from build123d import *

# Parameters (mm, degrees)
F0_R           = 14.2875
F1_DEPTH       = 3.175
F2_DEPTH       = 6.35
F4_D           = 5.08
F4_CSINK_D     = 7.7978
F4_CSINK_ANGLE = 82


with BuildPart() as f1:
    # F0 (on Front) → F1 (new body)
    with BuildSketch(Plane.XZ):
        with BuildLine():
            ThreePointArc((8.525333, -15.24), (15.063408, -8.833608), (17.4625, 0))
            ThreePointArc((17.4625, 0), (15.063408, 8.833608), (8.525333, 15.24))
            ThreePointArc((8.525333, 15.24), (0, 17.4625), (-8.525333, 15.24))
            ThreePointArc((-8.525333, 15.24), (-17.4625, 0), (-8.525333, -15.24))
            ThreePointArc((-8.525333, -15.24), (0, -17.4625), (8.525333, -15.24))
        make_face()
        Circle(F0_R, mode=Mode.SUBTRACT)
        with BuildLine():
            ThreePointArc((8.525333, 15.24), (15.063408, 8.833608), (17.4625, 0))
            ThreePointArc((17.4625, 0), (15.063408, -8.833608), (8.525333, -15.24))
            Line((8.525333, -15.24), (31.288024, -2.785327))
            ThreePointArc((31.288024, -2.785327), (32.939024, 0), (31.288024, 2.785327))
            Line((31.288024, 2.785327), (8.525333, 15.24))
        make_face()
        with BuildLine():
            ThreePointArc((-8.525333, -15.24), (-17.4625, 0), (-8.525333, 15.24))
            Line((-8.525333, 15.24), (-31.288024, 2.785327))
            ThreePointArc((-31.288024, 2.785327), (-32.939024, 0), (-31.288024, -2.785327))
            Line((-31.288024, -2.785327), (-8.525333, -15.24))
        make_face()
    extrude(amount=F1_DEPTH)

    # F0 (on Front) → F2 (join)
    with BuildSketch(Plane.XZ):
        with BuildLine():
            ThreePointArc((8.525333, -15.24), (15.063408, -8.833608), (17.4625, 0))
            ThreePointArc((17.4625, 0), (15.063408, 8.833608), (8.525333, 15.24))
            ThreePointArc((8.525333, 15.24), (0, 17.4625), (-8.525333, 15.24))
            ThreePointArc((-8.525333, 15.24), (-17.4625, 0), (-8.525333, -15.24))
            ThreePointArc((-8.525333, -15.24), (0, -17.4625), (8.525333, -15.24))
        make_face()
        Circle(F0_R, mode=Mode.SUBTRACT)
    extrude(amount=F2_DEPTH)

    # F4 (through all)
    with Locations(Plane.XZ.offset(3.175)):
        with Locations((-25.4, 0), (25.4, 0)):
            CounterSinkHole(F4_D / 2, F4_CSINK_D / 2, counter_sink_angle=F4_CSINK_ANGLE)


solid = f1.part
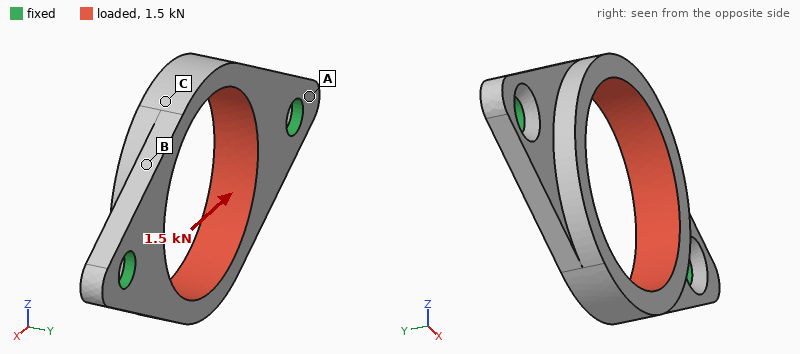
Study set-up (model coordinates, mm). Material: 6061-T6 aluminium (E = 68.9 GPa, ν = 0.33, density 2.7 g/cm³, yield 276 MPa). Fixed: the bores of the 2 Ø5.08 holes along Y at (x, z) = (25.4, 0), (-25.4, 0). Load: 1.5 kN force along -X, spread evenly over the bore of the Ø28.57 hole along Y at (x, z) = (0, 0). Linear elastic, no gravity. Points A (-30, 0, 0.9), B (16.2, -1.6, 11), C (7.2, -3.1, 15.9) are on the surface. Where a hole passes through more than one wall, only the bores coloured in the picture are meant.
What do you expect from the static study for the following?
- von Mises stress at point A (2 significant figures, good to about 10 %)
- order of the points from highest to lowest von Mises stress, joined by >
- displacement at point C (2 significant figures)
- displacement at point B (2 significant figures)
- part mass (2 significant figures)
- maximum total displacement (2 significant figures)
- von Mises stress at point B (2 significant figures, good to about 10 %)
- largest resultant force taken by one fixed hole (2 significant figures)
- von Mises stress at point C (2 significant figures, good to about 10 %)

8.2 MPa
B > C > A
12 µm
7.2 µm
8.8 g
13 µm
29 MPa
750 N
16 MPa
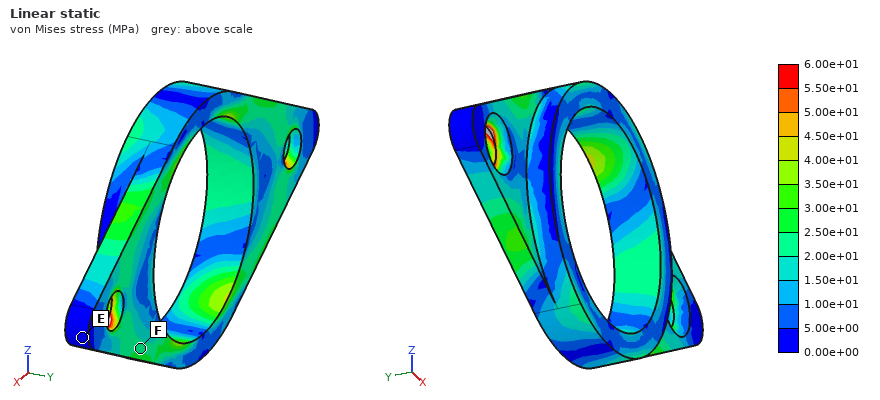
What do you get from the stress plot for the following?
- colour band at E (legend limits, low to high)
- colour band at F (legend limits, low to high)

0.00e+00 to 5.00e+00 MPa
2.00e+01 to 2.50e+01 MPa
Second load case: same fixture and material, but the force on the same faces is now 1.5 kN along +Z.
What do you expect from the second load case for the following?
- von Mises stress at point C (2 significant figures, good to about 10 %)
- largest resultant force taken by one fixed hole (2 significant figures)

18 MPa
750 N
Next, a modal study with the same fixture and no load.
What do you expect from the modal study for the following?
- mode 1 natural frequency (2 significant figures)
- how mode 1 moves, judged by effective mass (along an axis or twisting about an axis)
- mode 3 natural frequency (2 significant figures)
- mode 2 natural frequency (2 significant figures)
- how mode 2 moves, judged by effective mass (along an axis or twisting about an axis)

4700 Hz
twisting about X
14 kHz
6100 Hz
along Y
